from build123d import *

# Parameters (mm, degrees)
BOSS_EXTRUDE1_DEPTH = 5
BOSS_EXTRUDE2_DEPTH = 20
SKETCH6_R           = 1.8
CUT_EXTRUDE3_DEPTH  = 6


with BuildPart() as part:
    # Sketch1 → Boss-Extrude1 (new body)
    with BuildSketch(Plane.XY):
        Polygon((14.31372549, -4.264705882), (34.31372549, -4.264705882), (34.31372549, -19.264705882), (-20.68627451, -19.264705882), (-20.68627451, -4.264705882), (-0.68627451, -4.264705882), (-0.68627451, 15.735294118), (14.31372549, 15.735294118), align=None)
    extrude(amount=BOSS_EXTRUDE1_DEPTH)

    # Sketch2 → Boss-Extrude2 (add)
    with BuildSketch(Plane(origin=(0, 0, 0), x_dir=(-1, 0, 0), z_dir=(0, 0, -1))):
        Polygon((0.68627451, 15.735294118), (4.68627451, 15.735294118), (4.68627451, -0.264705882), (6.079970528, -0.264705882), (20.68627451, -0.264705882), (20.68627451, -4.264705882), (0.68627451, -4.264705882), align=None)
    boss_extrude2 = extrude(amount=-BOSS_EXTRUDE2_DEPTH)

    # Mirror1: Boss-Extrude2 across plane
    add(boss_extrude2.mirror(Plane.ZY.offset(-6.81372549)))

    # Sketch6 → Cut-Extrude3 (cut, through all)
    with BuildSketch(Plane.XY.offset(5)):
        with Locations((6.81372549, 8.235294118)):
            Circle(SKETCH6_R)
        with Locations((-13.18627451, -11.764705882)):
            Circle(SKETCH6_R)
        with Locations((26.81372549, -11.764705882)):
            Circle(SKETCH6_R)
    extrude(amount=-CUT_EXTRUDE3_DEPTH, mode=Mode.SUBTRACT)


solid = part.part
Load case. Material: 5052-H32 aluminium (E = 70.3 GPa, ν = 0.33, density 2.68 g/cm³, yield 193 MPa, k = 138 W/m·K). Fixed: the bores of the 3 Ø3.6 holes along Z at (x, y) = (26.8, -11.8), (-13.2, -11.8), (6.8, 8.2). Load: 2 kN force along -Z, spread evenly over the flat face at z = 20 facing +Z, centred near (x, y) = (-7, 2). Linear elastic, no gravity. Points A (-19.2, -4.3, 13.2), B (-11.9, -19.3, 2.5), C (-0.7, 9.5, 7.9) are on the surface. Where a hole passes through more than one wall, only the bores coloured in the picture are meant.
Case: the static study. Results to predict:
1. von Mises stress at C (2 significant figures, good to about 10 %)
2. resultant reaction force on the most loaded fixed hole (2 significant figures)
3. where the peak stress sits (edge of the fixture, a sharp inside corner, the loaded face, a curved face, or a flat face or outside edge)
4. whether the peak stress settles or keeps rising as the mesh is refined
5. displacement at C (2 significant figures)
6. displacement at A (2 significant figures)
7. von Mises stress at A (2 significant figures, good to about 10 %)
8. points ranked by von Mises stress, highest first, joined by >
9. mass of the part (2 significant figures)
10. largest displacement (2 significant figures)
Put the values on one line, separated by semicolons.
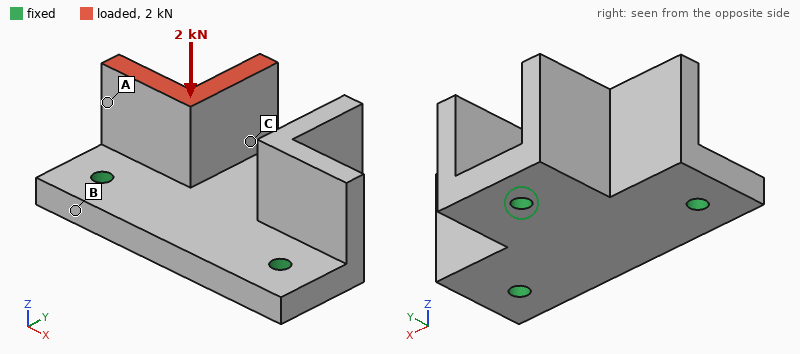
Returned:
38 MPa; 1.1 kN; edge of the fixture; keeps rising; 21 µm; 33 µm; 24 MPa; C > A > B; 30 g; 45 µm
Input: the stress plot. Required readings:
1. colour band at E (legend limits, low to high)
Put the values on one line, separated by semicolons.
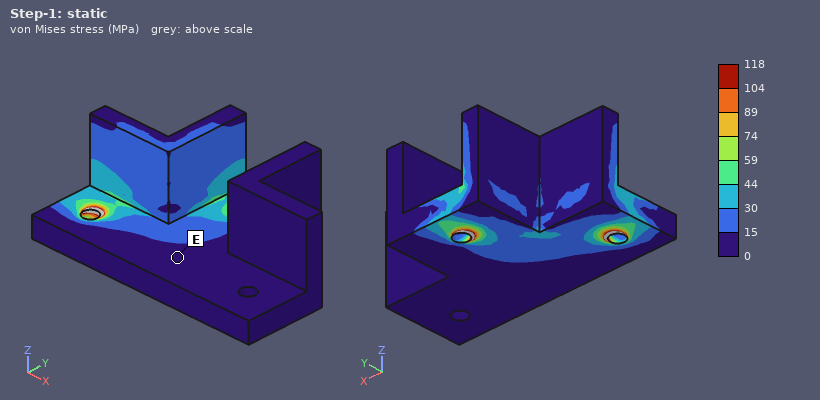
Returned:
0 to 15 MPa
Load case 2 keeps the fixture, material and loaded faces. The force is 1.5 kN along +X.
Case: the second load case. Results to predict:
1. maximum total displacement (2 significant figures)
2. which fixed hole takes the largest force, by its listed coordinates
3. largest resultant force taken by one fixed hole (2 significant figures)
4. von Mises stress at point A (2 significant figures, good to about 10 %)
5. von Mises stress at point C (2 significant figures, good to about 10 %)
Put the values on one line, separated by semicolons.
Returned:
0.15 mm; (-13.2, -11.8); 1.0 kN; 33 MPa; 82 MPa
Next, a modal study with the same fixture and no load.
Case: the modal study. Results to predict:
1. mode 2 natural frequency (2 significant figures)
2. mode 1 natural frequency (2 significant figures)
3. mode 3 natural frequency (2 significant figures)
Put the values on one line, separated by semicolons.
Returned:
11 kHz; 9900 Hz; 14 kHz
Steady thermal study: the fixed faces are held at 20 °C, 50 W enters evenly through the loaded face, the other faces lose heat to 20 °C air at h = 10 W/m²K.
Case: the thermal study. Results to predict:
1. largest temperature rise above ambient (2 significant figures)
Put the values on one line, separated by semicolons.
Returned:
58 K
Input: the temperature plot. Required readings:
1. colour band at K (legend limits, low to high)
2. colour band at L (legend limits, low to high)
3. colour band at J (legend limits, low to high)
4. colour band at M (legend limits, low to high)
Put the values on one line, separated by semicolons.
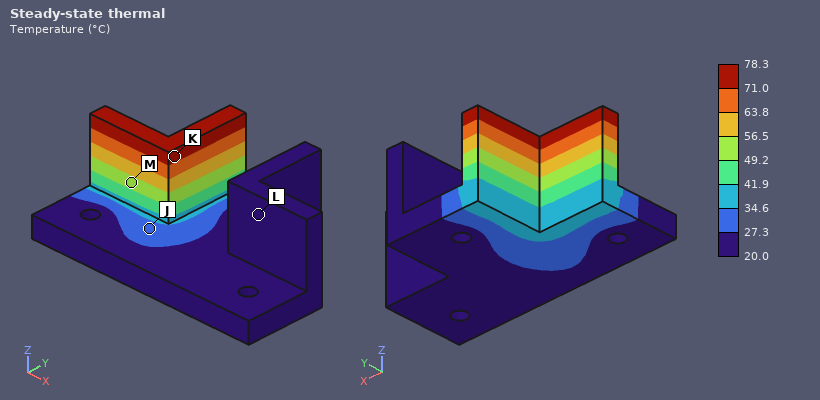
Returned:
71.0 to 78.3 °C; 20.0 to 27.3 °C; 27.3 to 34.6 °C; 49.2 to 56.5 °C
